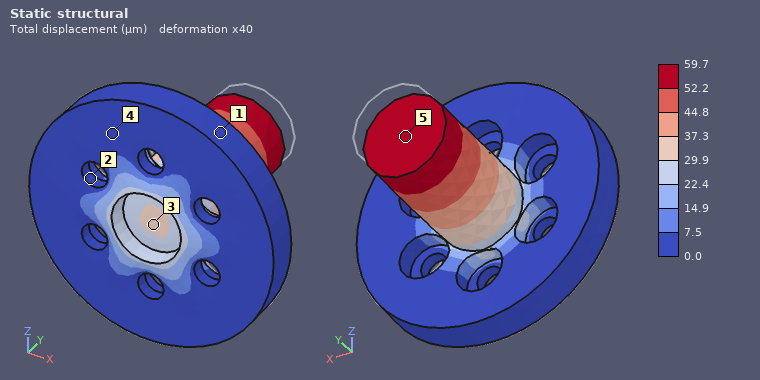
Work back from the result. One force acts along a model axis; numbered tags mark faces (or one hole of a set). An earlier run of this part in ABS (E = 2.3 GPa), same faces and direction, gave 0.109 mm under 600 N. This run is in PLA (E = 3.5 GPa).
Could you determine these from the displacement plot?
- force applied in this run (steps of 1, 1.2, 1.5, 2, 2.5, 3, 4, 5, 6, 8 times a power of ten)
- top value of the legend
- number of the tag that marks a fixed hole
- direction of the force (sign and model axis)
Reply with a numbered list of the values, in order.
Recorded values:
1. 500 N
2. 59.7 µm
3. 2
4. -Y
